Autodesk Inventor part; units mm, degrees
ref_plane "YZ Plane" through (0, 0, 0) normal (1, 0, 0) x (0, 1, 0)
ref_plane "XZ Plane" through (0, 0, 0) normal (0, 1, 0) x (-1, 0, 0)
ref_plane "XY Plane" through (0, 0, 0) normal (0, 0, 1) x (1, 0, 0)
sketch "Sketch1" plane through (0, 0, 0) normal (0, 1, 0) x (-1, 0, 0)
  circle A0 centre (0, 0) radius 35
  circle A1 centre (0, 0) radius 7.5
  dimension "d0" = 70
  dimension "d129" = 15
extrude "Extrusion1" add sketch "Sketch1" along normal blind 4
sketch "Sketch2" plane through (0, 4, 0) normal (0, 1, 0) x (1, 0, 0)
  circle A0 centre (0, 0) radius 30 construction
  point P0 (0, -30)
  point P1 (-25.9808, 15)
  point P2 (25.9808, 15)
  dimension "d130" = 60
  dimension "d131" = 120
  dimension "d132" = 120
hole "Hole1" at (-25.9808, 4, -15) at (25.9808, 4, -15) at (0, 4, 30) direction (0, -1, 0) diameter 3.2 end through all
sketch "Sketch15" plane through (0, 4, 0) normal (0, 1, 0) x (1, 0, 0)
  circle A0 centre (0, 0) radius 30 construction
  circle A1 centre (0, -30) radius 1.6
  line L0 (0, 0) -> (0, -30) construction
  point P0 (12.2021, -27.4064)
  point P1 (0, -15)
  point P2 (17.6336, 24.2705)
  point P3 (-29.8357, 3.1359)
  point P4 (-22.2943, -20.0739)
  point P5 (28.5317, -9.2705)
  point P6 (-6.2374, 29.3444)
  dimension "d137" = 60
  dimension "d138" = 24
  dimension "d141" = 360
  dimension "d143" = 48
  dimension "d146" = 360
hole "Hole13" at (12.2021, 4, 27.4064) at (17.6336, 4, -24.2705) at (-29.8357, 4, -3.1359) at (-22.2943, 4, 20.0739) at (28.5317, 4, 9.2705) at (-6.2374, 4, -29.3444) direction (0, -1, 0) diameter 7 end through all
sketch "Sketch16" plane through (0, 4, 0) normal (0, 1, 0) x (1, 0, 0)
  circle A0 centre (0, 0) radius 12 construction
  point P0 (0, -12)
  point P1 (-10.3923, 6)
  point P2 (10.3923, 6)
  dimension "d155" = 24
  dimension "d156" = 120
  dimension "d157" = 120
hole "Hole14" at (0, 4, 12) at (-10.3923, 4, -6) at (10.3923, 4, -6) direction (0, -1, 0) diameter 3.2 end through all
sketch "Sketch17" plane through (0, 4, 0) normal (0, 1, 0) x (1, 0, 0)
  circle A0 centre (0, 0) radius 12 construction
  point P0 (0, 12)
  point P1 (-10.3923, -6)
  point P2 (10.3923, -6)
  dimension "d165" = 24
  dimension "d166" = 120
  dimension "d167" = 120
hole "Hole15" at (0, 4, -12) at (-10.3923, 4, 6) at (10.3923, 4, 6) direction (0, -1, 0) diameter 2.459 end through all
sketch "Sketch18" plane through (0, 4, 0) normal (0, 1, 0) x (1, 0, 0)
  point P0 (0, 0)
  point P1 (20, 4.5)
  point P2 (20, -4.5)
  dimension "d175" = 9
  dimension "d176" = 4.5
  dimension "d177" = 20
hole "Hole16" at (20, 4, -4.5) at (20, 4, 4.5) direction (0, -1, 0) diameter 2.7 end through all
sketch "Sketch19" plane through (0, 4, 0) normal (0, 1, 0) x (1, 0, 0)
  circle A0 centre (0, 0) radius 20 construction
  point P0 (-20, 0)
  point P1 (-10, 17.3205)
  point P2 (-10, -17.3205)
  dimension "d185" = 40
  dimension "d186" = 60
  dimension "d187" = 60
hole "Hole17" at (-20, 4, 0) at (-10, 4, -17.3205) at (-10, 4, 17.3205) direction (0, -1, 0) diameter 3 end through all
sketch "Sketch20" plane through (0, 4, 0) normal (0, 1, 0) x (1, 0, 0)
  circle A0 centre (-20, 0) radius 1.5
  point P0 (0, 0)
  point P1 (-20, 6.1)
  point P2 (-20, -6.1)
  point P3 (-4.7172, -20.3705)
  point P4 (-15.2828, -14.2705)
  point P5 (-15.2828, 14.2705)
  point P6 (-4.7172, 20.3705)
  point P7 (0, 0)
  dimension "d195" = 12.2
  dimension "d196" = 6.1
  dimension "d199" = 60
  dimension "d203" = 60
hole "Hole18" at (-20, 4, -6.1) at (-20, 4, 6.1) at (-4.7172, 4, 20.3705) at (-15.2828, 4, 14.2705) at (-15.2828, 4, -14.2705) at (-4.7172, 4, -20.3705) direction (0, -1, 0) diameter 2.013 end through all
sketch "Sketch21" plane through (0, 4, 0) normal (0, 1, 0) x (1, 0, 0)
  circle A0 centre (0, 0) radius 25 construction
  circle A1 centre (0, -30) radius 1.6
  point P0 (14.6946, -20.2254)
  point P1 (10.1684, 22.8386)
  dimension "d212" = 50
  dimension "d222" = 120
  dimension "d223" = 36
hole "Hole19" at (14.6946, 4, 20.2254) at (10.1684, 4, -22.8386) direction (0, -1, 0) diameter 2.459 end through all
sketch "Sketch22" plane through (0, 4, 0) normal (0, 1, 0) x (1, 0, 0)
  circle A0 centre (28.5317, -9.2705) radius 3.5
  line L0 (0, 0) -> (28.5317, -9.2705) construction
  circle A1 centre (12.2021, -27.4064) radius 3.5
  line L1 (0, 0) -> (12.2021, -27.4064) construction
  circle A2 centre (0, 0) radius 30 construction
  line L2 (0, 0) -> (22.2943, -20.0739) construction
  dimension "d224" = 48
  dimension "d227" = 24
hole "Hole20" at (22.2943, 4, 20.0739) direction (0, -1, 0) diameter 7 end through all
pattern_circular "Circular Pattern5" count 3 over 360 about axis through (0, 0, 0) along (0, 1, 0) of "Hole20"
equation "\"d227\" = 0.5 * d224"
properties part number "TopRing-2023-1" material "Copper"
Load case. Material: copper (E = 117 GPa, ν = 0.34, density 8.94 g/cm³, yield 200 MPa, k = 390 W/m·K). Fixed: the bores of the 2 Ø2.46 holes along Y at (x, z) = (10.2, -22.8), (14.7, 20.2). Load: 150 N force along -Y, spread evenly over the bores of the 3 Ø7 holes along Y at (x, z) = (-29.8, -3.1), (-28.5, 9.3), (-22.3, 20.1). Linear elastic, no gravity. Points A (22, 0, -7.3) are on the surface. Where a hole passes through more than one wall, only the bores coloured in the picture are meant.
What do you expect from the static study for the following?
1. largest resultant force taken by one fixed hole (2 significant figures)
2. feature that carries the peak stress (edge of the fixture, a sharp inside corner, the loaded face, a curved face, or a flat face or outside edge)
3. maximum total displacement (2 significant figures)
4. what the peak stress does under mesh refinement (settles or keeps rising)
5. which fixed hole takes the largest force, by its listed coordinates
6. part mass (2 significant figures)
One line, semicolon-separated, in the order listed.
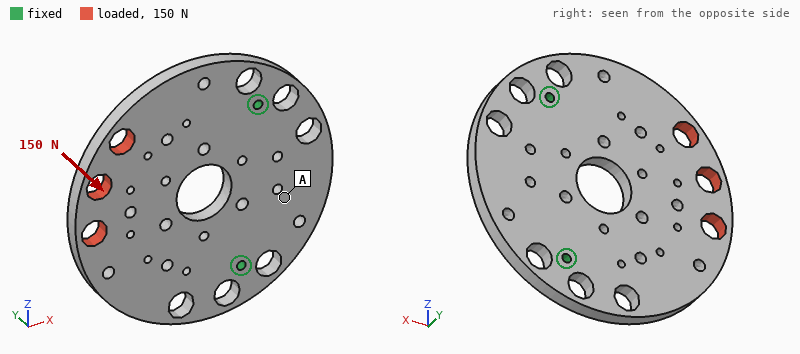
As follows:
95 N; edge of the fixture; 0.19 mm; keeps rising; (14.7, 20.2); 110 g
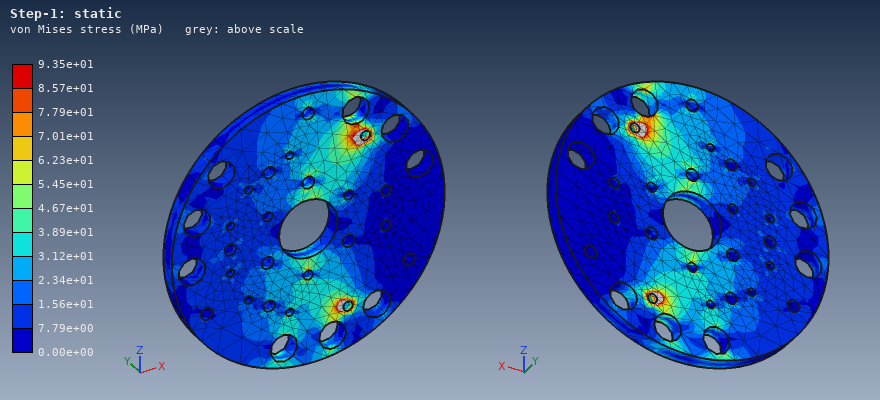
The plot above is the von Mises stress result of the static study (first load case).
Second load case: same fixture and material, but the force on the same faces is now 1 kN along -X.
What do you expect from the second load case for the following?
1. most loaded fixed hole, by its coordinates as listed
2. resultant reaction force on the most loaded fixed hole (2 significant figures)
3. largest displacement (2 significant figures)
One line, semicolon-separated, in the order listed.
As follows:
(14.7, 20.2); 740 N; 5.1 µm
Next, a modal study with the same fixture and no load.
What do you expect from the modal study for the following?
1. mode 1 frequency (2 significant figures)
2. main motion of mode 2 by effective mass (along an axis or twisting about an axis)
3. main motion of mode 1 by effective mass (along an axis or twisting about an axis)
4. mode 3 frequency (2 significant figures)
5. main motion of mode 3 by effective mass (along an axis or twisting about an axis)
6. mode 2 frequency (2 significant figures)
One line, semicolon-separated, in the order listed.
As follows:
1000 Hz; twisting about X; along Y; 3500 Hz; along Y; 2400 Hz
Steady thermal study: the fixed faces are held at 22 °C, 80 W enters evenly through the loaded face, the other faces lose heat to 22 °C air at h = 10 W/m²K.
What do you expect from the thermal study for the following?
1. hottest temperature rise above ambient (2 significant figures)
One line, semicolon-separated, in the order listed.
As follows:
64 K
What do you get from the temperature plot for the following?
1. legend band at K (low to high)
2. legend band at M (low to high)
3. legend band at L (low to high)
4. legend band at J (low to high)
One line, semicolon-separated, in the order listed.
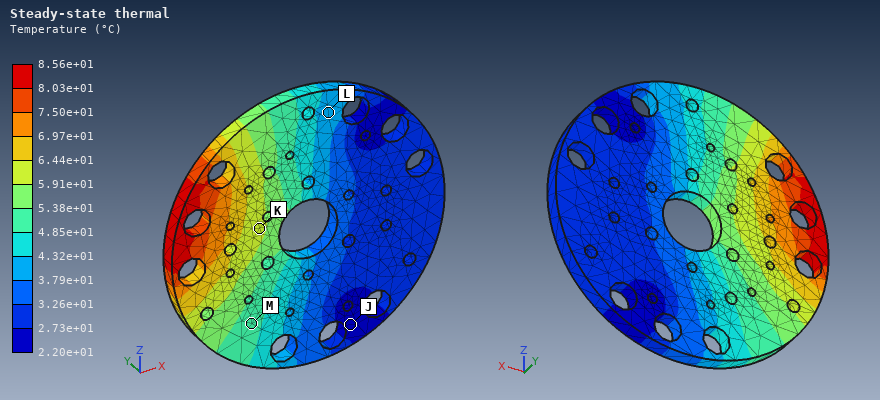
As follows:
5.91e+01 to 6.44e+01 °C; 4.85e+01 to 5.38e+01 °C; 3.79e+01 to 4.32e+01 °C; 2.20e+01 to 2.73e+01 °C
